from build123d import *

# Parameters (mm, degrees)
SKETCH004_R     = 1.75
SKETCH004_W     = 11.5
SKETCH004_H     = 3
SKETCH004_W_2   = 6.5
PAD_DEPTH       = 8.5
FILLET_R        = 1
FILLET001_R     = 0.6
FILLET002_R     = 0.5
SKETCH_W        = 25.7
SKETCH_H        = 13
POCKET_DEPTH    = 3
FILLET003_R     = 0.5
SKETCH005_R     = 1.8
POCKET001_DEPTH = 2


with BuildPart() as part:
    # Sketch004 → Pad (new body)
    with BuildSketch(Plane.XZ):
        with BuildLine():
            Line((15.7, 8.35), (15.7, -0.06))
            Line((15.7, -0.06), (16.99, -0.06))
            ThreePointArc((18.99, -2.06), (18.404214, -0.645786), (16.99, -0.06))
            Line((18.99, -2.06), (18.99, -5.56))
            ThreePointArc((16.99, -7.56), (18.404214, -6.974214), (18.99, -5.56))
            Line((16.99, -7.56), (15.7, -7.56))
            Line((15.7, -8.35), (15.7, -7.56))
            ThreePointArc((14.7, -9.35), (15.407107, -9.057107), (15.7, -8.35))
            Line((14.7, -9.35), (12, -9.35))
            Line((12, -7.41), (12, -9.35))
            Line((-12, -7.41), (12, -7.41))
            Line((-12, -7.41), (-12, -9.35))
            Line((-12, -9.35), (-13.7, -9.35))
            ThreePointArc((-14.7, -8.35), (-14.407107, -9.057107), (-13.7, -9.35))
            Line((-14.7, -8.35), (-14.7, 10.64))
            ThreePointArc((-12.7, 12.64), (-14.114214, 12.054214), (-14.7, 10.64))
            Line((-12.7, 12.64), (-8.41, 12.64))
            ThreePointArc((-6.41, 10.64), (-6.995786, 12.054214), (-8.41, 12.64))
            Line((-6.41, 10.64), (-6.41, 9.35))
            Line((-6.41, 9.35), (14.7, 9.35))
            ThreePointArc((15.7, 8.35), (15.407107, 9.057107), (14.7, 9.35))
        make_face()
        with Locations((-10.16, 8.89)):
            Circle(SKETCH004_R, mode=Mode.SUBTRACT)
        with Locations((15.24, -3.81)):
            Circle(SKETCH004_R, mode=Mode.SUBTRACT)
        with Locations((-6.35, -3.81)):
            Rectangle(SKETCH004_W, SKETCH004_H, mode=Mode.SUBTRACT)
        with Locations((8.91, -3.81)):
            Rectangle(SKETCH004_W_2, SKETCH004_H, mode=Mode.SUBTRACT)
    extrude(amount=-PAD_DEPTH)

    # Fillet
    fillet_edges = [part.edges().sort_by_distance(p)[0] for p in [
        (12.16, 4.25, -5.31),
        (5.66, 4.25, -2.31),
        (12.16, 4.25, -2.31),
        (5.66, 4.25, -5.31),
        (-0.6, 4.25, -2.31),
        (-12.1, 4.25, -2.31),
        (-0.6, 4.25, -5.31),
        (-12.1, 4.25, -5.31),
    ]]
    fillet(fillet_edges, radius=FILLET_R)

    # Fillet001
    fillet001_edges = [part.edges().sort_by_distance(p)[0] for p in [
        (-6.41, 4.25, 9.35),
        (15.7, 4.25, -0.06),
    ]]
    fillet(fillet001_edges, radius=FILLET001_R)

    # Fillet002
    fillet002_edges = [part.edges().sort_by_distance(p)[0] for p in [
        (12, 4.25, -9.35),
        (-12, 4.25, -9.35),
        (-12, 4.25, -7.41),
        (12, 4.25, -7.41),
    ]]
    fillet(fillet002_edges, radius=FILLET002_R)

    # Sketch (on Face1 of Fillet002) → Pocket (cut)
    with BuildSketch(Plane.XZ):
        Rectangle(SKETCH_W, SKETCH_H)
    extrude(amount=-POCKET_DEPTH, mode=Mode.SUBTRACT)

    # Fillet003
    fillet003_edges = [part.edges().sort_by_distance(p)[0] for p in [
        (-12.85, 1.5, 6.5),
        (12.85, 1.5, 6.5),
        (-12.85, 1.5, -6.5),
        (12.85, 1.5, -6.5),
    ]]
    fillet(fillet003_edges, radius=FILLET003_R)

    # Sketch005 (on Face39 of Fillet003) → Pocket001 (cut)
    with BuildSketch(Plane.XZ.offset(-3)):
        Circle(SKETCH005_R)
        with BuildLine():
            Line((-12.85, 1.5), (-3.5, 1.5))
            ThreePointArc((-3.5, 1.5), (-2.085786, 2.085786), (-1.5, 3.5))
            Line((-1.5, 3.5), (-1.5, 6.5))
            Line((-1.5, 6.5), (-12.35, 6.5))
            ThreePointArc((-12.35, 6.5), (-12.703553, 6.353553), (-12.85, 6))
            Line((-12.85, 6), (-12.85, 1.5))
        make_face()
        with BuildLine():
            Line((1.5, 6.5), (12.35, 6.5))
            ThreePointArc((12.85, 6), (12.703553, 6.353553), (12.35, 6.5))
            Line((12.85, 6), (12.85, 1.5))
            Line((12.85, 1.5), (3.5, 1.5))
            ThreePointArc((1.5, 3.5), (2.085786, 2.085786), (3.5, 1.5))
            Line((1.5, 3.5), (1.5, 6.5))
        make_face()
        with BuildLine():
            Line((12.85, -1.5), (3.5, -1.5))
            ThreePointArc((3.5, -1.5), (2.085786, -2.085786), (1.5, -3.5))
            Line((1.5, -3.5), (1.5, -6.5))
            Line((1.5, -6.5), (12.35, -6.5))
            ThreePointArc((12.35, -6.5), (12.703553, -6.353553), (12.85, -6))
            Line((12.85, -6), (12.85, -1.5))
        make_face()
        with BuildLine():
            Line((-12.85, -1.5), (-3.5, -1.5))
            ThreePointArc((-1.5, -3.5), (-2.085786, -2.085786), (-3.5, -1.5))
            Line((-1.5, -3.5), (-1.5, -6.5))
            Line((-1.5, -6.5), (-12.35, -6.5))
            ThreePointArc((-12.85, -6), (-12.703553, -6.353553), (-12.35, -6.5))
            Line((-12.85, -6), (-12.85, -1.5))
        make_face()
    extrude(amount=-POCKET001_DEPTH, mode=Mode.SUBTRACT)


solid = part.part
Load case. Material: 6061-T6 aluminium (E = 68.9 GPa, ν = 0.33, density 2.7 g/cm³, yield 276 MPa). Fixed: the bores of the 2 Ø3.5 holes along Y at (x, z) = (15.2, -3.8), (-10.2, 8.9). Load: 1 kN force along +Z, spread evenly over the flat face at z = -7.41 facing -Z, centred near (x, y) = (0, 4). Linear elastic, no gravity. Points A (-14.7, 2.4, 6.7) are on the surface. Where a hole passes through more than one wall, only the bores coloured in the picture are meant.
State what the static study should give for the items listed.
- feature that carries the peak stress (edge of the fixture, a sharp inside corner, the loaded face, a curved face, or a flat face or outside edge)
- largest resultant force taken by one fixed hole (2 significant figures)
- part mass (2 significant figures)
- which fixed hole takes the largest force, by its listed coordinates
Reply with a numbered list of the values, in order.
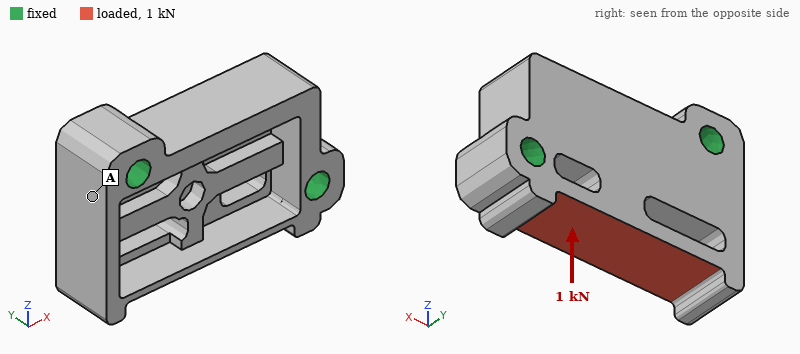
1. the loaded face
2. 600 N
3. 8.2 g
4. (-10.2, 8.9)
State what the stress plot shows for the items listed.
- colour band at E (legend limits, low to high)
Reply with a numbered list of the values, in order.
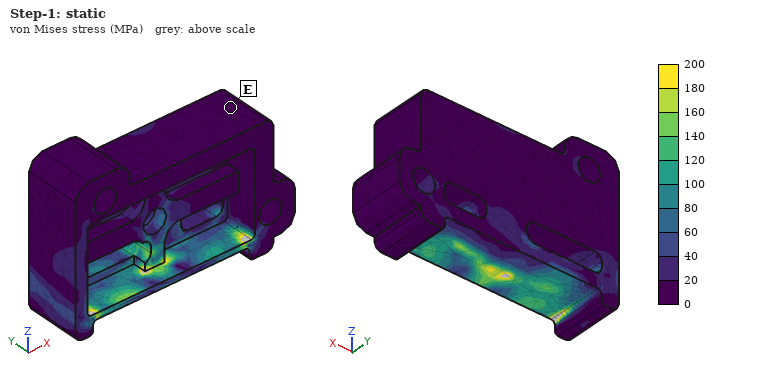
1. 0 to 20 MPa
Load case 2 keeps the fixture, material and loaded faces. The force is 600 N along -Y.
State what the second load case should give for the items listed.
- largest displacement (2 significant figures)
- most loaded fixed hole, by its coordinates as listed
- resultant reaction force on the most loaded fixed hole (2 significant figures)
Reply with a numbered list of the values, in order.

1. 46 µm
2. (15.2, -3.8)
3. 380 N
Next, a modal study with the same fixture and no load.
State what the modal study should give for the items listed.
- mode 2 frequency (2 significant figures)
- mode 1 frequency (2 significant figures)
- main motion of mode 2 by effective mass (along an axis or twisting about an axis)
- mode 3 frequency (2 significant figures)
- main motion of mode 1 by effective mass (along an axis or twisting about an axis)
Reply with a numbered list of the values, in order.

1. 27 kHz
2. 17 kHz
3. along Y
4. 30 kHz
5. along Y
